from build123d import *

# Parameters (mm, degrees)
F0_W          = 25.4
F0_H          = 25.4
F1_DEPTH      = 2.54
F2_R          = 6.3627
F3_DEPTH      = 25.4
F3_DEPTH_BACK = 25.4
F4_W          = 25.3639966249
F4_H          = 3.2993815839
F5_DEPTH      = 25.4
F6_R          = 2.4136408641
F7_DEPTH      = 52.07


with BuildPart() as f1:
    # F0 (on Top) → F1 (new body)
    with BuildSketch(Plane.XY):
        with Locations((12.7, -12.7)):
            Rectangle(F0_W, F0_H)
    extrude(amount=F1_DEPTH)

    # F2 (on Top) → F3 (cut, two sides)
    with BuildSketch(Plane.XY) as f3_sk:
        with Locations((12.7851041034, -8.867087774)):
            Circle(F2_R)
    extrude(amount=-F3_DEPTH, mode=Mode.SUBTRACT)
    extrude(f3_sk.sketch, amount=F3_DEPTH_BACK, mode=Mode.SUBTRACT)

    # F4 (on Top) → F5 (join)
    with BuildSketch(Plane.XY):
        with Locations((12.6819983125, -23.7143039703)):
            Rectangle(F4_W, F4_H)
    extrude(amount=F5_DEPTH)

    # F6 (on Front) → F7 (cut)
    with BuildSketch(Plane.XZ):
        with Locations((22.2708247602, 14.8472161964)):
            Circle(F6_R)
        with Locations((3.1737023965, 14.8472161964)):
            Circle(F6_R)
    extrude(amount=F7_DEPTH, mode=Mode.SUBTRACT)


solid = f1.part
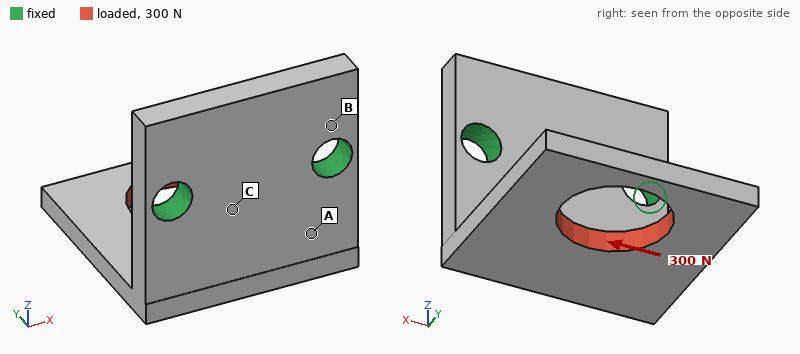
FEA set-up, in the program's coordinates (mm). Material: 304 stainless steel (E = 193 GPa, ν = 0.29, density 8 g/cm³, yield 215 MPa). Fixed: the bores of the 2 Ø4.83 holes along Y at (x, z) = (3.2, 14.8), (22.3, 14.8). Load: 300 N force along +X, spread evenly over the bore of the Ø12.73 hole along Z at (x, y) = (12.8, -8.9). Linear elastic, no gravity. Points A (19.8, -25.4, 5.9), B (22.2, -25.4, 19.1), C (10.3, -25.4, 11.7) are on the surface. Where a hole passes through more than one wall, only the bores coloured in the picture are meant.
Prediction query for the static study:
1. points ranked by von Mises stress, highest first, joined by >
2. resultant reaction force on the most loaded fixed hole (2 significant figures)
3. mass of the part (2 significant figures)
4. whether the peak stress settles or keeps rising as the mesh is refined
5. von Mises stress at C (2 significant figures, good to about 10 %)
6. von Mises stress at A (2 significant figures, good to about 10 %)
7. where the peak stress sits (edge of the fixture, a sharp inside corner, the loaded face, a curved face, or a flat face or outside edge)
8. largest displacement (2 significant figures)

A > C > B
330 N
25 g
keeps rising
17 MPa
40 MPa
edge of the fixture
36 µm
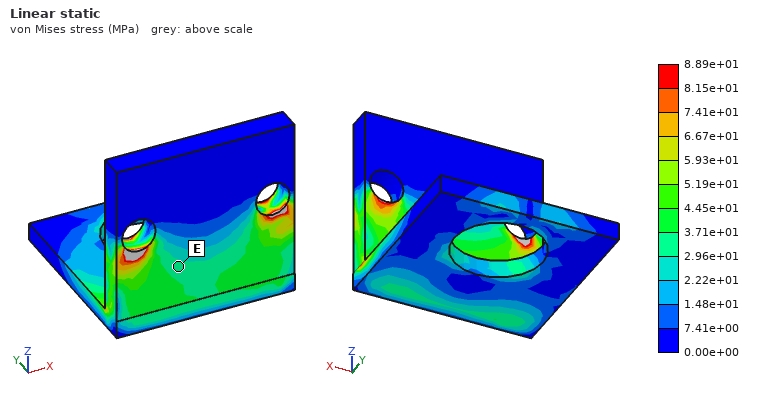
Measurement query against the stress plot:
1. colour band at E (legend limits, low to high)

2.96e+01 to 3.71e+01 MPa
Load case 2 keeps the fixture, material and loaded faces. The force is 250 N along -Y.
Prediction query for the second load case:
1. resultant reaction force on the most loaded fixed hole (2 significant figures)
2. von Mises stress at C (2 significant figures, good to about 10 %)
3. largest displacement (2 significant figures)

130 N
32 MPa
34 µm
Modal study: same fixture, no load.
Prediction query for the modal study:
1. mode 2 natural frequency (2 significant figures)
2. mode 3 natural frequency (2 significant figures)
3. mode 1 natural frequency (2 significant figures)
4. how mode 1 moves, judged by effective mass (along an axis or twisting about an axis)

5700 Hz
7400 Hz
2800 Hz
along Z
